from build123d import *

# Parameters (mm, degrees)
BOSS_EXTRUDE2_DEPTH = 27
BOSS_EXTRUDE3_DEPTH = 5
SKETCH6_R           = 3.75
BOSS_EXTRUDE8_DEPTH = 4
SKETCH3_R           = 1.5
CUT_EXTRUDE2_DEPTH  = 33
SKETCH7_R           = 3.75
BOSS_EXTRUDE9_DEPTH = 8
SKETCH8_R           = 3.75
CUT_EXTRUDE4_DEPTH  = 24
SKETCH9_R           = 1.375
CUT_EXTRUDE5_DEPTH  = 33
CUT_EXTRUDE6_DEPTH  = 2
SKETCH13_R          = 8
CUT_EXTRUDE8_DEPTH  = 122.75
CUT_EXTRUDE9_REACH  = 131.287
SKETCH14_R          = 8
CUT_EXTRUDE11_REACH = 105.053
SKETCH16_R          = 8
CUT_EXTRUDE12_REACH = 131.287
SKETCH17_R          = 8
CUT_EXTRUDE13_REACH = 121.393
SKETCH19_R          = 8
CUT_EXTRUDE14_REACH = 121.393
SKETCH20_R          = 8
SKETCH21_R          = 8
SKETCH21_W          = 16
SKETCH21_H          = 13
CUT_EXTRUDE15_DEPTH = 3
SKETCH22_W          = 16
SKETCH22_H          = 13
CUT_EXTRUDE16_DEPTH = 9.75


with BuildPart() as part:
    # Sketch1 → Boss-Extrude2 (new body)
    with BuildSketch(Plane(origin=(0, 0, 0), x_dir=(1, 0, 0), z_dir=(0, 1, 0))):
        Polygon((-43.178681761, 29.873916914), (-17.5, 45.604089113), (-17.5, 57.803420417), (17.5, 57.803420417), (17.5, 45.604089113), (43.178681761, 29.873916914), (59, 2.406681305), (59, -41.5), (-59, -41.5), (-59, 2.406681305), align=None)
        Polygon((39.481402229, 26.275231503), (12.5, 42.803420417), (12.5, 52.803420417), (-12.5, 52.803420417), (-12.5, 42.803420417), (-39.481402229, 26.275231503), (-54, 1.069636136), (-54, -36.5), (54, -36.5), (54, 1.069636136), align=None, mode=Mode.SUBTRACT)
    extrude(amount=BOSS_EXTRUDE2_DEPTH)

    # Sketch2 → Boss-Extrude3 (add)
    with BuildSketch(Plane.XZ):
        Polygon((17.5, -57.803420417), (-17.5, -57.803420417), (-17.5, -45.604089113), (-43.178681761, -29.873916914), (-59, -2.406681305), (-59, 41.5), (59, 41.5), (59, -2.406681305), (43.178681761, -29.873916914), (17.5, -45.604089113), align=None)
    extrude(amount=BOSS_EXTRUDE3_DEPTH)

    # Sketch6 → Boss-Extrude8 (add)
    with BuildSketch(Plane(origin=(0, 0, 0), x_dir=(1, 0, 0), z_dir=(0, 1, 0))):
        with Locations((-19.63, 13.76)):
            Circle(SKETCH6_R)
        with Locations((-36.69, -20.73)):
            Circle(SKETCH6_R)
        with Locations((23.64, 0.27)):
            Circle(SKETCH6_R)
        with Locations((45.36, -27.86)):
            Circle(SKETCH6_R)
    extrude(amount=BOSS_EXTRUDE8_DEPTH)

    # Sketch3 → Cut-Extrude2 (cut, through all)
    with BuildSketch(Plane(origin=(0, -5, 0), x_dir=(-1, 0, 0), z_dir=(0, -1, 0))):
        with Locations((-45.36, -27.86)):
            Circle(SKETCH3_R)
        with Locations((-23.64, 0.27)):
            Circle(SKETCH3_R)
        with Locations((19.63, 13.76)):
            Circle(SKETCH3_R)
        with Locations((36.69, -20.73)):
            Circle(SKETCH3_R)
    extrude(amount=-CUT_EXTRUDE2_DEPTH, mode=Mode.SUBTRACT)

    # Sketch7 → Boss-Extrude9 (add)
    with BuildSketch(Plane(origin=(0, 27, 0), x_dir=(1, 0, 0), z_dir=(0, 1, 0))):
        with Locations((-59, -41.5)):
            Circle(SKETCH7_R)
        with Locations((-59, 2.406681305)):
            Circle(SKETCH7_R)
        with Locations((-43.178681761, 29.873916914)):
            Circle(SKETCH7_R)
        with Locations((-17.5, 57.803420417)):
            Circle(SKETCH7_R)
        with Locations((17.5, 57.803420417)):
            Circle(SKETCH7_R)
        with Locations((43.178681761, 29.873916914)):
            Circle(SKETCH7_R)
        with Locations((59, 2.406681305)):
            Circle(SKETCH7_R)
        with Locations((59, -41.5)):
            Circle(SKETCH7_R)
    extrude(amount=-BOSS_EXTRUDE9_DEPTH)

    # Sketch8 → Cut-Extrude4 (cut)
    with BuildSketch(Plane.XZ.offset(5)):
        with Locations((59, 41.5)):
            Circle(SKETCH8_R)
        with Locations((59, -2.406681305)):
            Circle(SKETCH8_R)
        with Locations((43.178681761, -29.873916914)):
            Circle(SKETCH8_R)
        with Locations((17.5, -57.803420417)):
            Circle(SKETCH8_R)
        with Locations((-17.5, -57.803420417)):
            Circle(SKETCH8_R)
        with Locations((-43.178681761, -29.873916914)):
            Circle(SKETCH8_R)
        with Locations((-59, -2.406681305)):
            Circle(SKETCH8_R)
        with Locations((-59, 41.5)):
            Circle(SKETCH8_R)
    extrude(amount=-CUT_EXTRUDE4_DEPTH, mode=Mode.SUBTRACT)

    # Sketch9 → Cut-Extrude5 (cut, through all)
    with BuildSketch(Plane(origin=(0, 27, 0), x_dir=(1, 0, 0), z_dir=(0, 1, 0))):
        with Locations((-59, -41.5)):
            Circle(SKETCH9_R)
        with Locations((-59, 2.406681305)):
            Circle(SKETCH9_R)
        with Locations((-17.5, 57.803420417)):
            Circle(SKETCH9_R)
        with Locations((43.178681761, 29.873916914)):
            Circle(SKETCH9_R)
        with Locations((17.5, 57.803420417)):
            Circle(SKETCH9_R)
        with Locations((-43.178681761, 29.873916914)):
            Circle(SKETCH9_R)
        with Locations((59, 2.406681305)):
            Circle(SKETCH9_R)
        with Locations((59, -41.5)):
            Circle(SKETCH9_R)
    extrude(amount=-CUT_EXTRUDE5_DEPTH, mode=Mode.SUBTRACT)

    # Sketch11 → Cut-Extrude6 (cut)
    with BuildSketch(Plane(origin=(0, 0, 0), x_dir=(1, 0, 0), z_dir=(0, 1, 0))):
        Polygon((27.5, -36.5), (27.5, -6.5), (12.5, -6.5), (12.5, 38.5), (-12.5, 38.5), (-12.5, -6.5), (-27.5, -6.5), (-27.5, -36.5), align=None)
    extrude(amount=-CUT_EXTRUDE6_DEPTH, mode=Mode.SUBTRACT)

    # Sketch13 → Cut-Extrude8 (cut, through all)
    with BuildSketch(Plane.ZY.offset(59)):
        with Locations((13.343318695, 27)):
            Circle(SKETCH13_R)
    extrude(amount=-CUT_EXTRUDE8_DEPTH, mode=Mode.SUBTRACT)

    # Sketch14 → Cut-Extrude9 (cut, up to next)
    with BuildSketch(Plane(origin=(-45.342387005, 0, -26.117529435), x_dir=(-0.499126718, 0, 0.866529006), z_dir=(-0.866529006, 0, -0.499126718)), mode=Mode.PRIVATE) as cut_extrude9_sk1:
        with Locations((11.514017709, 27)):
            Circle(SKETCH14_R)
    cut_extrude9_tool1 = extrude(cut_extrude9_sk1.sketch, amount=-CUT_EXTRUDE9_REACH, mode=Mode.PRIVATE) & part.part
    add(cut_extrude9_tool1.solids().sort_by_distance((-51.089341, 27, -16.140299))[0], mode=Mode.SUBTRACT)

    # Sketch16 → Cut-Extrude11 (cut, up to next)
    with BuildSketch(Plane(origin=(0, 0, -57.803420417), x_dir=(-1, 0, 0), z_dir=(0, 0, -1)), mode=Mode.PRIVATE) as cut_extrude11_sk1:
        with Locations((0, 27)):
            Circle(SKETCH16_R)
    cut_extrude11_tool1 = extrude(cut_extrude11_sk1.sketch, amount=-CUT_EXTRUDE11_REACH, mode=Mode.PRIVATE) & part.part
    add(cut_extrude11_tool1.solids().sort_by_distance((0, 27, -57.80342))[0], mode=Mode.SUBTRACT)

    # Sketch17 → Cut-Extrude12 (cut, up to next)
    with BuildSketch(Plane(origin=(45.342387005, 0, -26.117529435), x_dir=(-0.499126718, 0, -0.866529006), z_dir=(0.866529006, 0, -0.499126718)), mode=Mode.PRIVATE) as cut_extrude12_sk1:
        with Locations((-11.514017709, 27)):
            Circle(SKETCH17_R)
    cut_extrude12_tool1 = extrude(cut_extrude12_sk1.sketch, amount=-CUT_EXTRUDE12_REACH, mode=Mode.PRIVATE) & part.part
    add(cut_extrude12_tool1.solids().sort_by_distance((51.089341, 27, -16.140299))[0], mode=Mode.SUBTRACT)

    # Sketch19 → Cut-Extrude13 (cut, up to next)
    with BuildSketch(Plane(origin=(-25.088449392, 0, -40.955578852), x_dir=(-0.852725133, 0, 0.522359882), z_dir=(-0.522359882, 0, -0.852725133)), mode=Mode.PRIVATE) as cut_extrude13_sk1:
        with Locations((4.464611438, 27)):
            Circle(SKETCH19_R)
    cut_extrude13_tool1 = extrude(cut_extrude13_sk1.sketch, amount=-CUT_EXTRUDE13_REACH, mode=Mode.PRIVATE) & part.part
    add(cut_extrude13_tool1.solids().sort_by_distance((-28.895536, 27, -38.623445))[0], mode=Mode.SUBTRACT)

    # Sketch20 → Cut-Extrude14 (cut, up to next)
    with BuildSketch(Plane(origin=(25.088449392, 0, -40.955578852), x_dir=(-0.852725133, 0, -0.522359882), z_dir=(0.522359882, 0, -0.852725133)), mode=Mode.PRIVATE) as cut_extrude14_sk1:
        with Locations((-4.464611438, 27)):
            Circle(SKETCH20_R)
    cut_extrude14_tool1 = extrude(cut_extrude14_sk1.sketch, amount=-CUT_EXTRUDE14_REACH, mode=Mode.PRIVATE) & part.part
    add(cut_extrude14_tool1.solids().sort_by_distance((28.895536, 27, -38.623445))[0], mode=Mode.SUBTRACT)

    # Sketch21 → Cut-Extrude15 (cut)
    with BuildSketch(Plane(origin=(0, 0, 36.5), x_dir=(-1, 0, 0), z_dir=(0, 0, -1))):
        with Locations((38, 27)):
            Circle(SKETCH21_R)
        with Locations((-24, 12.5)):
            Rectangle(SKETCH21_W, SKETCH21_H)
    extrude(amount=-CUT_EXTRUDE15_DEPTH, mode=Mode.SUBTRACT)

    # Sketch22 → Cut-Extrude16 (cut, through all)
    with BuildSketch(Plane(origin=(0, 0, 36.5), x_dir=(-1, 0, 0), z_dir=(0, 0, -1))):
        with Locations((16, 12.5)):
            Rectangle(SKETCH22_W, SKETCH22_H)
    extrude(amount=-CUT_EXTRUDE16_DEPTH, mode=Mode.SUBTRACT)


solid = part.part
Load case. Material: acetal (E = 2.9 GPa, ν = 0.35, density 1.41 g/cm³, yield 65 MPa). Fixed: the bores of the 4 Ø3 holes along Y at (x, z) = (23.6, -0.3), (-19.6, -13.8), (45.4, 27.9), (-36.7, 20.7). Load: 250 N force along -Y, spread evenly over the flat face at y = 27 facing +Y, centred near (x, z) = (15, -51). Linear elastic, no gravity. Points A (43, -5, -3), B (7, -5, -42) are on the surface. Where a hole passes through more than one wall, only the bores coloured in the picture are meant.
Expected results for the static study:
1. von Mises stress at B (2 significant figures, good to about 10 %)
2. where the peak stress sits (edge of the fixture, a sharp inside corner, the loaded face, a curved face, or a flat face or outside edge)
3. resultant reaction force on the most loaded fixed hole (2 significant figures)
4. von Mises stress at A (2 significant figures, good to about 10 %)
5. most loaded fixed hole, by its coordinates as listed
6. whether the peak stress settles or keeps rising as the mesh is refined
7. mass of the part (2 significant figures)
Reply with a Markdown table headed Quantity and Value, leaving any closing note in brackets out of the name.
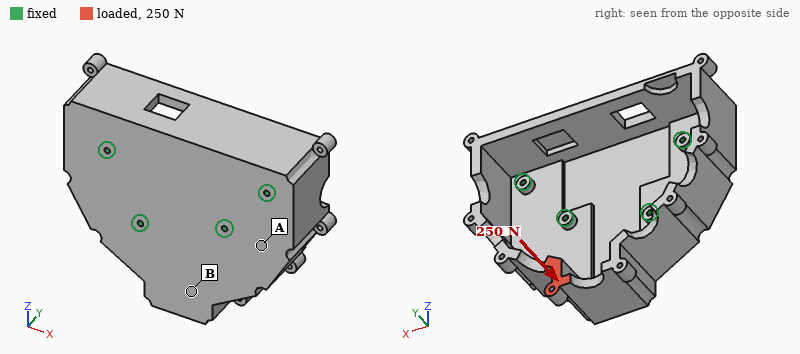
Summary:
| Quantity | Value |
|---|---|
| von Mises stress at B | 2.0 MPa |
| where the peak stress sits | edge of the fixture |
| resultant reaction force on the most loaded fixed hole | 260 N |
| von Mises stress at A | 5.7 MPa |
| most loaded fixed hole, by its coordinates as listed | (-19.6, -13.8) |
| whether the peak stress settles or keeps rising as the mesh is refined | keeps rising |
| mass of the part | 120 g |
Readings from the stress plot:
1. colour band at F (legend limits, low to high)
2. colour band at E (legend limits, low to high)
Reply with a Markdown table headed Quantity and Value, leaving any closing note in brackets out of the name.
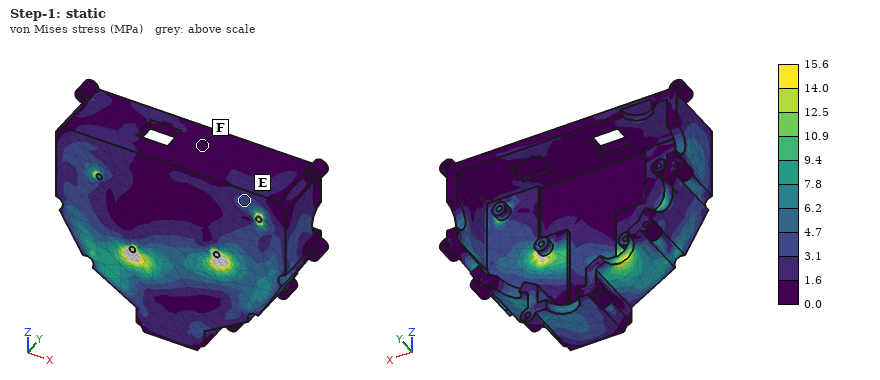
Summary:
| Quantity | Value |
|---|---|
| colour band at F | 0.0 to 1.6 MPa |
| colour band at E | 3.1 to 4.7 MPa |
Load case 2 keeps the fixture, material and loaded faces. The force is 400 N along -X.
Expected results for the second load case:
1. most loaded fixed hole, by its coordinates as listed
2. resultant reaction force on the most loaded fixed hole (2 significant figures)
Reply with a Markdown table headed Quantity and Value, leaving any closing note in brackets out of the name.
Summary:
| Quantity | Value |
|---|---|
| most loaded fixed hole, by its coordinates as listed | (-19.6, -13.8) |
| resultant reaction force on the most loaded fixed hole | 300 N |
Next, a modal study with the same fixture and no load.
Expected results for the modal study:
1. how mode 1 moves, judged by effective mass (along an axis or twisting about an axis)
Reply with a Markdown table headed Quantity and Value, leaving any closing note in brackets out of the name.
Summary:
| Quantity | Value |
|---|---|
| how mode 1 moves, judged by effective mass | along Y |
